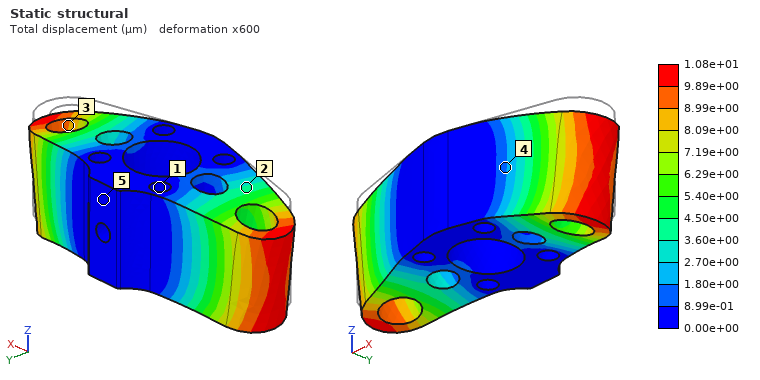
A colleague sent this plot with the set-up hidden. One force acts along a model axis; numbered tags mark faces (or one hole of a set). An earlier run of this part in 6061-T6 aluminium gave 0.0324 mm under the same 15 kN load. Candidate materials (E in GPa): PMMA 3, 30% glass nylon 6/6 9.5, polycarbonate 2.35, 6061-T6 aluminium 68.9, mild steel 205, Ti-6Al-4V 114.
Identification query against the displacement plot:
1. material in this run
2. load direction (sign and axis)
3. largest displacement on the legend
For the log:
mild steel
-Z
1.08e+01 µm
